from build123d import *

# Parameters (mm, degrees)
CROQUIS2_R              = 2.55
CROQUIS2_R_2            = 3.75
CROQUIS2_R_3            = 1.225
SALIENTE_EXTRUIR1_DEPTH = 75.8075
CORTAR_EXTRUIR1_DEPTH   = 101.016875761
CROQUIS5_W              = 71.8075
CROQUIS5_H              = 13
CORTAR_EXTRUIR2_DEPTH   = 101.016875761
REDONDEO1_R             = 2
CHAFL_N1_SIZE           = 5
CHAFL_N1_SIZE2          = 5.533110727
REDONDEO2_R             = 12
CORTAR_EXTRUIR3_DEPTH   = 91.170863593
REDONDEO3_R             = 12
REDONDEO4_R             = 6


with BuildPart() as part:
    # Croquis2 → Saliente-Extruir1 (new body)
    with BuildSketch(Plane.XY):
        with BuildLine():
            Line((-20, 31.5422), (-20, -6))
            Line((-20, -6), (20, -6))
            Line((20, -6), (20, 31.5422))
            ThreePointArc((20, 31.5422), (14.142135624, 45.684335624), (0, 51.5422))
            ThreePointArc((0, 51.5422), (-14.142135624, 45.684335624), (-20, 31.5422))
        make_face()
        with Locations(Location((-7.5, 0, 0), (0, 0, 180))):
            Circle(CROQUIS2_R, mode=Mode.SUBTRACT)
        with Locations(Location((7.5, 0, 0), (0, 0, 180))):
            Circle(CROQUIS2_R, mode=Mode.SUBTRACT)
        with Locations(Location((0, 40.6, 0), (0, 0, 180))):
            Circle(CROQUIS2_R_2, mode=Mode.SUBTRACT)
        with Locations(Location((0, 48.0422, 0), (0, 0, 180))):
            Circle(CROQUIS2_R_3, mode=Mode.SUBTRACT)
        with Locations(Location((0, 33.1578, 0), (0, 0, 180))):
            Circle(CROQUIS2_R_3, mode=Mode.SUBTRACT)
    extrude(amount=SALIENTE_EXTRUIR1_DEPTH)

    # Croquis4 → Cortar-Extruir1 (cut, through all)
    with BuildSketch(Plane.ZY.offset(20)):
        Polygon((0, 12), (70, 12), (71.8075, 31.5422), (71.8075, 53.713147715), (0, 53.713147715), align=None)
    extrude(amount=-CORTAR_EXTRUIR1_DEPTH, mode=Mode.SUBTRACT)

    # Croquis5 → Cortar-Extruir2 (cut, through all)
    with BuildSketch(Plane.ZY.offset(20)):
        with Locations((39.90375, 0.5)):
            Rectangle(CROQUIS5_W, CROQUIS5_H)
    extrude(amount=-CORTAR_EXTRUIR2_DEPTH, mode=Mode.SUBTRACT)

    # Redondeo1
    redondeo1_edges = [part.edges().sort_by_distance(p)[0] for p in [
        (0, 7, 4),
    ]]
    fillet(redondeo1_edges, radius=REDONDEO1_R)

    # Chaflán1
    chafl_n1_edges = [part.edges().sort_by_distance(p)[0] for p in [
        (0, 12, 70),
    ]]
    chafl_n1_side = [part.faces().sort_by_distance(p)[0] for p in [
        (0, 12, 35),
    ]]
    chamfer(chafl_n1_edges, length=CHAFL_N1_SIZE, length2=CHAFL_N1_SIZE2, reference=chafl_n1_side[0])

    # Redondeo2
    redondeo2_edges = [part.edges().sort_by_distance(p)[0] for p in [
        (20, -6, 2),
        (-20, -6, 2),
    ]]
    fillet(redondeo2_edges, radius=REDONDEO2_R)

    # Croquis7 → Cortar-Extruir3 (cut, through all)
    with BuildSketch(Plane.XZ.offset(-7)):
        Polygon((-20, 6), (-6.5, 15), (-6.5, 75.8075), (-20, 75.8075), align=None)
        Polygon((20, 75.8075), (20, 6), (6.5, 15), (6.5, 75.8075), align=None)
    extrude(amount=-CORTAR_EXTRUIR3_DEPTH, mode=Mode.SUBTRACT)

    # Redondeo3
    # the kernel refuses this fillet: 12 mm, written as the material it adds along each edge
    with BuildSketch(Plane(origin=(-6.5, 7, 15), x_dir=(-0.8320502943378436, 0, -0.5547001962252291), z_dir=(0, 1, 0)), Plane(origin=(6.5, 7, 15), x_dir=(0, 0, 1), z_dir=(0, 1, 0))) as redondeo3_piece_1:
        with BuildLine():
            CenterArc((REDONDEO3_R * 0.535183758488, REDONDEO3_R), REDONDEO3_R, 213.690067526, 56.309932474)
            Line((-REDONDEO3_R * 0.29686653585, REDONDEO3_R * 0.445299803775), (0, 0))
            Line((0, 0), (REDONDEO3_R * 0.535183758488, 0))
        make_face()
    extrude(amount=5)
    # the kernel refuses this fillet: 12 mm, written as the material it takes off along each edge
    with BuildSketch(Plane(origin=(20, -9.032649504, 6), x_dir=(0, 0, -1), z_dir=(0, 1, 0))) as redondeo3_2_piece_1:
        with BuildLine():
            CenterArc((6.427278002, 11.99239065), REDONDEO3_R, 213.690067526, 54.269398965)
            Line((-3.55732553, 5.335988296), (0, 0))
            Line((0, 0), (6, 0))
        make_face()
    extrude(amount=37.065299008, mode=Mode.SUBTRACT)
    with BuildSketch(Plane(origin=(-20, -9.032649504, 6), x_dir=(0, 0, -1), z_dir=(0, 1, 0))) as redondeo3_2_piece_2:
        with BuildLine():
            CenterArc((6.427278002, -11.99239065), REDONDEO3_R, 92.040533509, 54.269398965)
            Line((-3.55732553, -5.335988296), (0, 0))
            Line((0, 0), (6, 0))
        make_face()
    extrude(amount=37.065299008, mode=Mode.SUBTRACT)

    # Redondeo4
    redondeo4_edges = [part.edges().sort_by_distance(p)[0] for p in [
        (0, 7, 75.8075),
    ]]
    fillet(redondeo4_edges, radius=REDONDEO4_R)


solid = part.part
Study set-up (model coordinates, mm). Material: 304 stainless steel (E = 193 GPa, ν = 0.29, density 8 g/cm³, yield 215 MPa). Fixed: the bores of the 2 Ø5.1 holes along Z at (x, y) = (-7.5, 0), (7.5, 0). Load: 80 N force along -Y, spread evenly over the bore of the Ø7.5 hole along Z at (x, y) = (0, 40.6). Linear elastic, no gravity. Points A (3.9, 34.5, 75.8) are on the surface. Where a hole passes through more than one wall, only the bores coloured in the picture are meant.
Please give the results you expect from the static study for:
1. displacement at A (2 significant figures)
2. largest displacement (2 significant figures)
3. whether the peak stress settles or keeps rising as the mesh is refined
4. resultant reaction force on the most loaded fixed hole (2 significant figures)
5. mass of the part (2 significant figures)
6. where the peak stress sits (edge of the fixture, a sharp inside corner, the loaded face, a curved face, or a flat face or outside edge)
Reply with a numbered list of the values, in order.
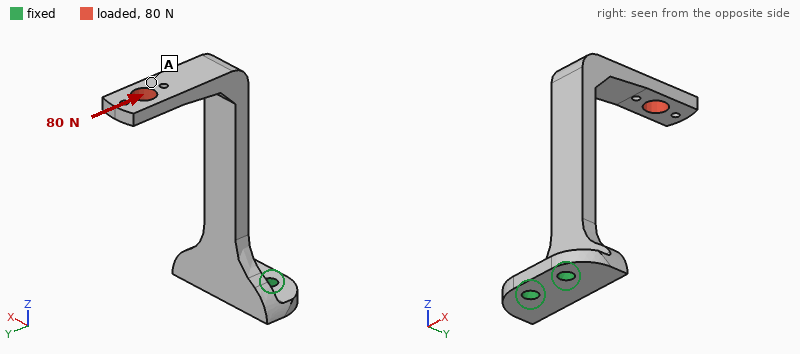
1. 0.42 mm
2. 0.50 mm
3. keeps rising
4. 59 N
5. 81 g
6. edge of the fixture
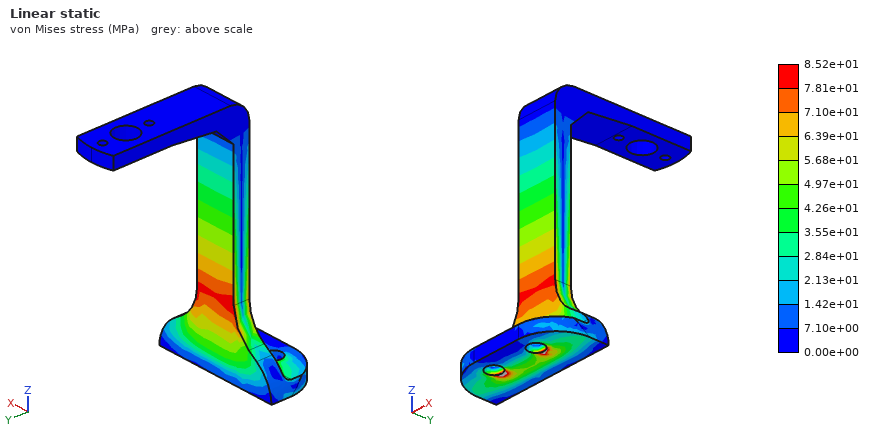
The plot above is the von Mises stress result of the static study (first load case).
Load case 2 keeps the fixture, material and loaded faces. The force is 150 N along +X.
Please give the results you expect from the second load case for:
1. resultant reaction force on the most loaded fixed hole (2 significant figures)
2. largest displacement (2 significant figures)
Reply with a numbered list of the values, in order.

1. 640 N
2. 0.42 mm
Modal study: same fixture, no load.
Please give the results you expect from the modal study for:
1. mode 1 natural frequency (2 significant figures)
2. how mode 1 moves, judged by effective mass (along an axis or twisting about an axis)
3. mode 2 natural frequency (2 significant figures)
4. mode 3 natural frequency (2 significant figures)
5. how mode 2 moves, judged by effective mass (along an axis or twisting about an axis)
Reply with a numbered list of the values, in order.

1. 430 Hz
2. along Y
3. 1000 Hz
4. 1900 Hz
5. along X
